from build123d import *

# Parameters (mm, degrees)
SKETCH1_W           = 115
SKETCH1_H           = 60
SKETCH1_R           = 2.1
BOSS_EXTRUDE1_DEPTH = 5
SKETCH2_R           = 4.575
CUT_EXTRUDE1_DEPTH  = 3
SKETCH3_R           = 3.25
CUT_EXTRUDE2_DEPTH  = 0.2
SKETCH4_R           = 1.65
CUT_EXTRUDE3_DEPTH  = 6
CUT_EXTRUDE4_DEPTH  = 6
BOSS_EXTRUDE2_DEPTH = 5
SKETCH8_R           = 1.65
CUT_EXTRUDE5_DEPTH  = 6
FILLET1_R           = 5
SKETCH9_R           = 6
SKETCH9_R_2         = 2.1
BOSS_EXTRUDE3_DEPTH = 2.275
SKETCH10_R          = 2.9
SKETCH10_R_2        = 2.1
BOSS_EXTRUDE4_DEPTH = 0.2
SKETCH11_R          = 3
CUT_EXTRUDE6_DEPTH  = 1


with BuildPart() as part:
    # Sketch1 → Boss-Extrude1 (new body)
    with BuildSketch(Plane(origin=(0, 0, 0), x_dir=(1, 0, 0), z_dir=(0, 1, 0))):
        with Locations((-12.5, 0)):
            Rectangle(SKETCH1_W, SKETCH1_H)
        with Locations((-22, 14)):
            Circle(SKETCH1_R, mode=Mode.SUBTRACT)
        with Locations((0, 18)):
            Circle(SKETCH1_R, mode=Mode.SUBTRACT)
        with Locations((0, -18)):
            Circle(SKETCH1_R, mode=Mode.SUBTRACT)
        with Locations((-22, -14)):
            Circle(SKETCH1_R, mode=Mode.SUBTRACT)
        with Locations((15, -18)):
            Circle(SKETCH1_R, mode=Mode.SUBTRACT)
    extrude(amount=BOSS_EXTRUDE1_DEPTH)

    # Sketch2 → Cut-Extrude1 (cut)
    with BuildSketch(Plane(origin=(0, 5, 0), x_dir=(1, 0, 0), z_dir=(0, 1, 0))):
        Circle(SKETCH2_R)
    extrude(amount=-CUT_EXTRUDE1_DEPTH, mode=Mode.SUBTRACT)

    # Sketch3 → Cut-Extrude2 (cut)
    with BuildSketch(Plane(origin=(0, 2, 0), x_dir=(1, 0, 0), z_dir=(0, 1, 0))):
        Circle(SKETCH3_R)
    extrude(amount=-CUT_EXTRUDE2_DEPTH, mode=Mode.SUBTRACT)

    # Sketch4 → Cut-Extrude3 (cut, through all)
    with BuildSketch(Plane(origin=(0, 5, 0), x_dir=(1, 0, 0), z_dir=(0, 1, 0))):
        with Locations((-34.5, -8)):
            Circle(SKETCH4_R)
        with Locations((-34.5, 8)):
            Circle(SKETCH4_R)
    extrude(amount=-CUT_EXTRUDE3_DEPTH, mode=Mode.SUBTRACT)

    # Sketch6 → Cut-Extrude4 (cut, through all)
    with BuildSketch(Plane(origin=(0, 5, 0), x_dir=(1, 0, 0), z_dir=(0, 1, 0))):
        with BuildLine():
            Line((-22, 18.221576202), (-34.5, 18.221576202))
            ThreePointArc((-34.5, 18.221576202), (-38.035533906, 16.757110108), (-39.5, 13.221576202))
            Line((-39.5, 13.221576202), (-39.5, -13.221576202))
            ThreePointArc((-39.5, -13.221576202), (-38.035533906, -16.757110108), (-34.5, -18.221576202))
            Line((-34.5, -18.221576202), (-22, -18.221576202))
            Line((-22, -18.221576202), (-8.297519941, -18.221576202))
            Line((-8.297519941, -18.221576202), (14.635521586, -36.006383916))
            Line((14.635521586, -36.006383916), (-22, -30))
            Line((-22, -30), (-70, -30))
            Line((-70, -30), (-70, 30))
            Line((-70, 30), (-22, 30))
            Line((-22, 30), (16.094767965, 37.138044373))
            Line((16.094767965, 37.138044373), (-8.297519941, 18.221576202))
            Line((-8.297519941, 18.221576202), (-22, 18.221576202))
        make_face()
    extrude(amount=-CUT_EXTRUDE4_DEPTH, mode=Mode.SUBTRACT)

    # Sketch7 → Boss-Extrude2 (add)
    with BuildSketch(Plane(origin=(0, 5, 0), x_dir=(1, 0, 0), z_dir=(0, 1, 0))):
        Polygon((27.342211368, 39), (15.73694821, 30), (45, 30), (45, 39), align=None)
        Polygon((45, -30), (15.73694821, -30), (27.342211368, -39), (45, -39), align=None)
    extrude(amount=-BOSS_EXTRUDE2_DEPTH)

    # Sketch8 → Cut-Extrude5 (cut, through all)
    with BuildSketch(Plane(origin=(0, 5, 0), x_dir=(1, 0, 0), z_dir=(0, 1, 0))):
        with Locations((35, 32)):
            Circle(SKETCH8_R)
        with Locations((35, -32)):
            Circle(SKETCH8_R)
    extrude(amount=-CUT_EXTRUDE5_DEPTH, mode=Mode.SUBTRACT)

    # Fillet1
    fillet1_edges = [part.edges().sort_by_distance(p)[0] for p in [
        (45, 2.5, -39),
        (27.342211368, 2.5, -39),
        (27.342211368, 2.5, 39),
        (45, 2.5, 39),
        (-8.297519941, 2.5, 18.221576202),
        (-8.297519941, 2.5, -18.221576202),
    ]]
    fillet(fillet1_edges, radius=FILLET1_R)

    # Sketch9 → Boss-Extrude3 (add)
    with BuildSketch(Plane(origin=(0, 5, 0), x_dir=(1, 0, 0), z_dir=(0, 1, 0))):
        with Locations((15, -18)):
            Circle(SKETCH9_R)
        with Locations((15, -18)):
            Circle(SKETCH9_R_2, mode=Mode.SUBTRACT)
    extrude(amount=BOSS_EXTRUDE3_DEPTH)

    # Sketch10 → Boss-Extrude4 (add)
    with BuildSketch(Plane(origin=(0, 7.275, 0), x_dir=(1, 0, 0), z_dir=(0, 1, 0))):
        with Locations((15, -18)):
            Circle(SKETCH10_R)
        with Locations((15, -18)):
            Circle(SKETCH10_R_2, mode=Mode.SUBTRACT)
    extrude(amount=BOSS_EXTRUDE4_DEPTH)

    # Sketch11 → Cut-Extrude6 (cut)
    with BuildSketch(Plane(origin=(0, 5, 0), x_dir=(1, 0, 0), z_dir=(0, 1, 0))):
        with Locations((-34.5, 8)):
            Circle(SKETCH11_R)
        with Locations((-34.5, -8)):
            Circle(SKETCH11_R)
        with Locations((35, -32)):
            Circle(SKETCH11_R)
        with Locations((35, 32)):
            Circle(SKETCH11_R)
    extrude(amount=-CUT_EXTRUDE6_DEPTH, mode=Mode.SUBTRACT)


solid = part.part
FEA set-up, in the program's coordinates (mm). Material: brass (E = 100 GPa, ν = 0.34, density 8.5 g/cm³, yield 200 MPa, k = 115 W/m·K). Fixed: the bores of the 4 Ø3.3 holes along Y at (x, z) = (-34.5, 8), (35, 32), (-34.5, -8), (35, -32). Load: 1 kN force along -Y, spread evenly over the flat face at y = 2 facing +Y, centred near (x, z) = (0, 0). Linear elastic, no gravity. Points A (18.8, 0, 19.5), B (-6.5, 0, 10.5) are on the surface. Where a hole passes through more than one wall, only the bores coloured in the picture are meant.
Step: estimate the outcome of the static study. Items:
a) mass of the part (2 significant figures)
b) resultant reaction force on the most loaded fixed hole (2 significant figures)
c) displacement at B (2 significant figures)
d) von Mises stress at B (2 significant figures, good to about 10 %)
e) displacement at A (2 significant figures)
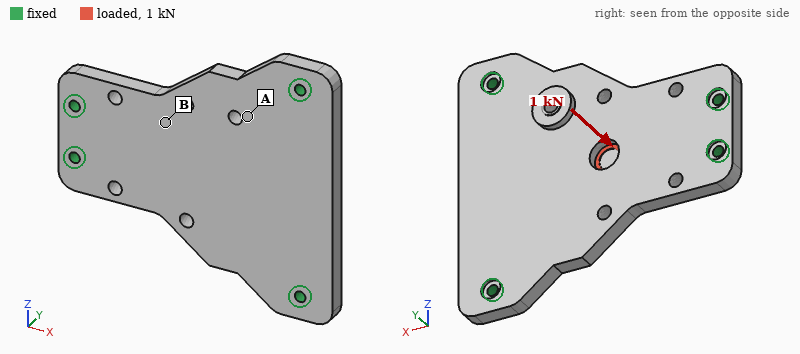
190 g
270 N
56 µm
38 MPa
33 µm
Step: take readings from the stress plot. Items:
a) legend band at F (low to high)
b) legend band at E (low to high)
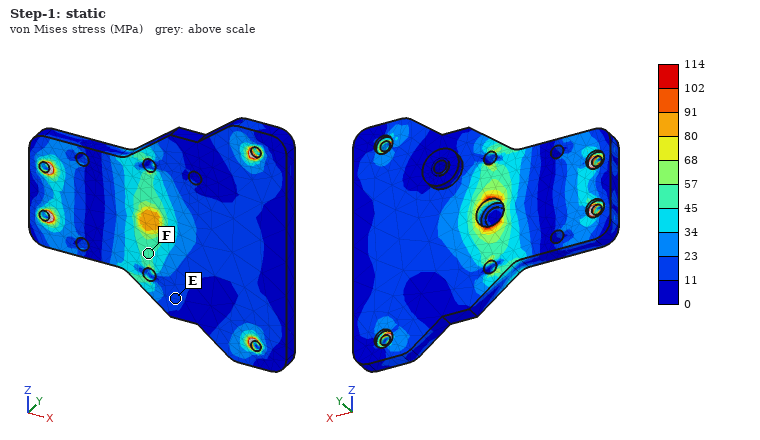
45 to 57 MPa
11 to 23 MPa
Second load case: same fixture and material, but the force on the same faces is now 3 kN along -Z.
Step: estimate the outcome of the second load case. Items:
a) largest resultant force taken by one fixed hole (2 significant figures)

1.3 kN
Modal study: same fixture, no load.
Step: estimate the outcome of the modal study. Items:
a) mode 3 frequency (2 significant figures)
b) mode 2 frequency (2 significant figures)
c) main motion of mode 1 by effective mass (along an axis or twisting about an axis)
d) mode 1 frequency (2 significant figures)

4200 Hz
4100 Hz
along Y
2500 Hz
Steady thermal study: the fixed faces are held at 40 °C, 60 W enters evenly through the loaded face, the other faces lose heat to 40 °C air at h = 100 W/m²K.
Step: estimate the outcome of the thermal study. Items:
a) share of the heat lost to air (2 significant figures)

31 %
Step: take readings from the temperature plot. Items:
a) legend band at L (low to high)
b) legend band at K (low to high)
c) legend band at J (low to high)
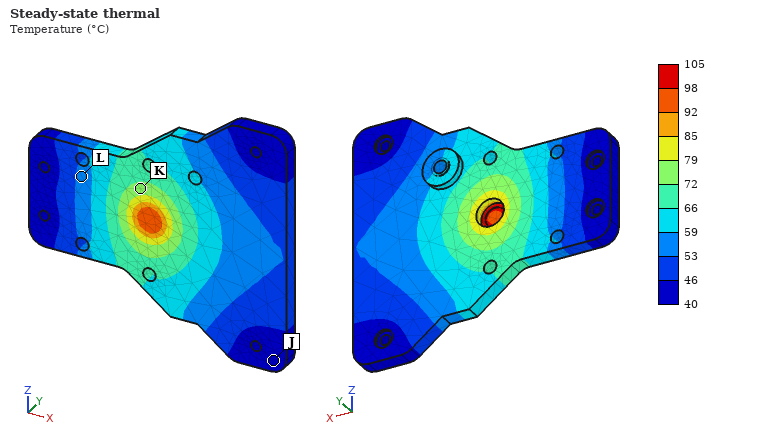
53 to 59 °C
72 to 79 °C
40 to 46 °C
